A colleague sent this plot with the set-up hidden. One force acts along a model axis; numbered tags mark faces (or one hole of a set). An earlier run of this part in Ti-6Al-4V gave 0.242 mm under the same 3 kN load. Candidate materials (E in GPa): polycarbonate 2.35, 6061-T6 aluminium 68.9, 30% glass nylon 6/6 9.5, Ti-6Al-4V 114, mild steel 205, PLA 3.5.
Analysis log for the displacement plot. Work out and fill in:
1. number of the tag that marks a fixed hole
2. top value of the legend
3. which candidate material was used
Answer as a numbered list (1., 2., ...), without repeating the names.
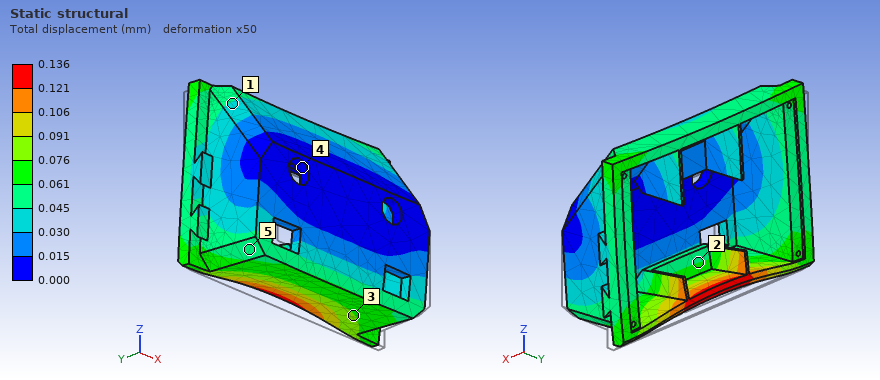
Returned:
1. 4
2. 0.136 mm
3. mild steel
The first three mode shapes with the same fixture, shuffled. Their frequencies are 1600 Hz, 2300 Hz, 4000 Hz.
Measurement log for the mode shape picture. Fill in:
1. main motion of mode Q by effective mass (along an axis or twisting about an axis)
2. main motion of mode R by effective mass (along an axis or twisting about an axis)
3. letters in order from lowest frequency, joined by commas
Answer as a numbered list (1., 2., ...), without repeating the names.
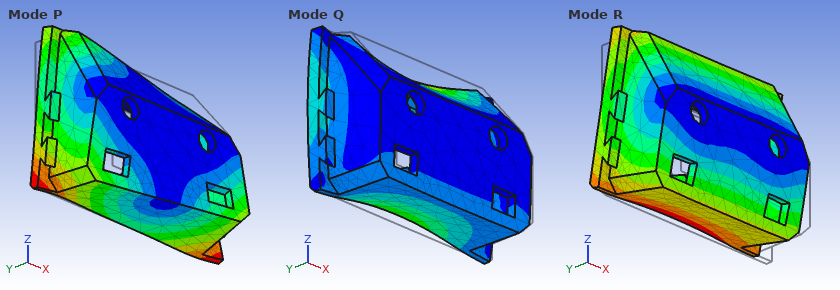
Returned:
1. along Y
2. along Z
3. R, P, Q
